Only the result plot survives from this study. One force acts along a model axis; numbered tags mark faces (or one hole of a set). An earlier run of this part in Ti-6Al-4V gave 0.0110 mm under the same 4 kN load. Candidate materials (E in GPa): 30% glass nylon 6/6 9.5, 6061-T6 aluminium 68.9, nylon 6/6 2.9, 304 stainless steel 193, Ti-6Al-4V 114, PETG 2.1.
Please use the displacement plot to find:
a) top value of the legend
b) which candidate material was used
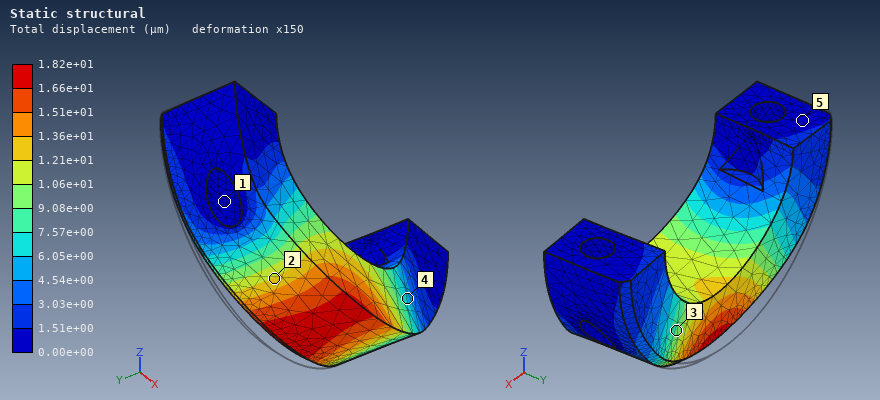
1.82e+01 µm
6061-T6 aluminium
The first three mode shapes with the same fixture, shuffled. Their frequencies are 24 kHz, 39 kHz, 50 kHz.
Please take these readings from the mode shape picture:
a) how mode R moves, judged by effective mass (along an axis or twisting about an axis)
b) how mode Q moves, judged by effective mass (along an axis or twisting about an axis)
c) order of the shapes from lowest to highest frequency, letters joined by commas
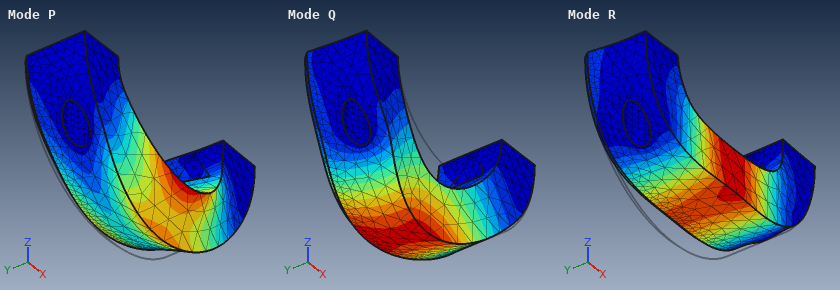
along Z
along Y
Q, R, P
